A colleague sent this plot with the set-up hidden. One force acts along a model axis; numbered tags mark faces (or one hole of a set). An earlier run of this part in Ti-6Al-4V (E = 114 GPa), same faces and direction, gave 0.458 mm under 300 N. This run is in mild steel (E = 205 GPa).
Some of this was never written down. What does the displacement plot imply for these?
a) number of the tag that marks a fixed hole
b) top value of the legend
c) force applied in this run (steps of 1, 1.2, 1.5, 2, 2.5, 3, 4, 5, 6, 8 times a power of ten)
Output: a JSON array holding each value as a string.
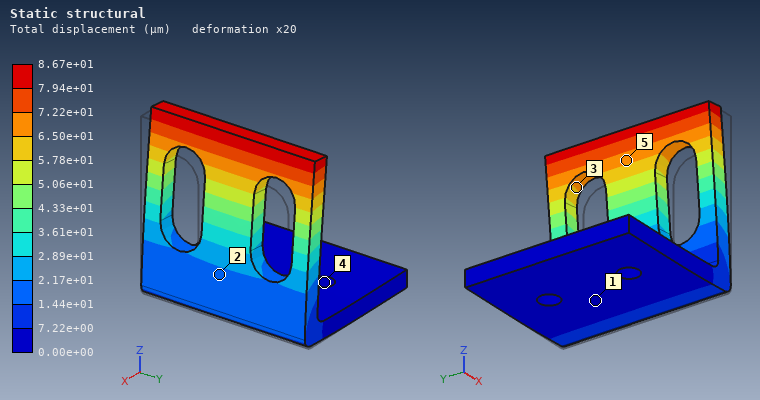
["4", "8.67e+01 µm", "100 N"]
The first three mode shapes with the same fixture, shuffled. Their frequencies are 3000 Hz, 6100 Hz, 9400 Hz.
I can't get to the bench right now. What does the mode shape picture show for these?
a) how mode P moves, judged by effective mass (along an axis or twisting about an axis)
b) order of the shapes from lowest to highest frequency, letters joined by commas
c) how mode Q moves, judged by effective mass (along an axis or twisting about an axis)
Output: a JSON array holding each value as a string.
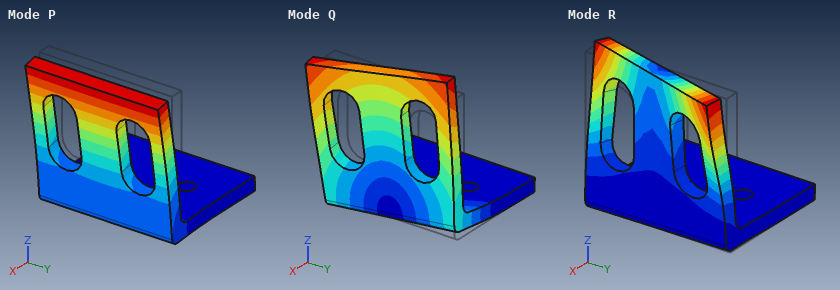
["along X", "P, Q, R", "along Y"]
